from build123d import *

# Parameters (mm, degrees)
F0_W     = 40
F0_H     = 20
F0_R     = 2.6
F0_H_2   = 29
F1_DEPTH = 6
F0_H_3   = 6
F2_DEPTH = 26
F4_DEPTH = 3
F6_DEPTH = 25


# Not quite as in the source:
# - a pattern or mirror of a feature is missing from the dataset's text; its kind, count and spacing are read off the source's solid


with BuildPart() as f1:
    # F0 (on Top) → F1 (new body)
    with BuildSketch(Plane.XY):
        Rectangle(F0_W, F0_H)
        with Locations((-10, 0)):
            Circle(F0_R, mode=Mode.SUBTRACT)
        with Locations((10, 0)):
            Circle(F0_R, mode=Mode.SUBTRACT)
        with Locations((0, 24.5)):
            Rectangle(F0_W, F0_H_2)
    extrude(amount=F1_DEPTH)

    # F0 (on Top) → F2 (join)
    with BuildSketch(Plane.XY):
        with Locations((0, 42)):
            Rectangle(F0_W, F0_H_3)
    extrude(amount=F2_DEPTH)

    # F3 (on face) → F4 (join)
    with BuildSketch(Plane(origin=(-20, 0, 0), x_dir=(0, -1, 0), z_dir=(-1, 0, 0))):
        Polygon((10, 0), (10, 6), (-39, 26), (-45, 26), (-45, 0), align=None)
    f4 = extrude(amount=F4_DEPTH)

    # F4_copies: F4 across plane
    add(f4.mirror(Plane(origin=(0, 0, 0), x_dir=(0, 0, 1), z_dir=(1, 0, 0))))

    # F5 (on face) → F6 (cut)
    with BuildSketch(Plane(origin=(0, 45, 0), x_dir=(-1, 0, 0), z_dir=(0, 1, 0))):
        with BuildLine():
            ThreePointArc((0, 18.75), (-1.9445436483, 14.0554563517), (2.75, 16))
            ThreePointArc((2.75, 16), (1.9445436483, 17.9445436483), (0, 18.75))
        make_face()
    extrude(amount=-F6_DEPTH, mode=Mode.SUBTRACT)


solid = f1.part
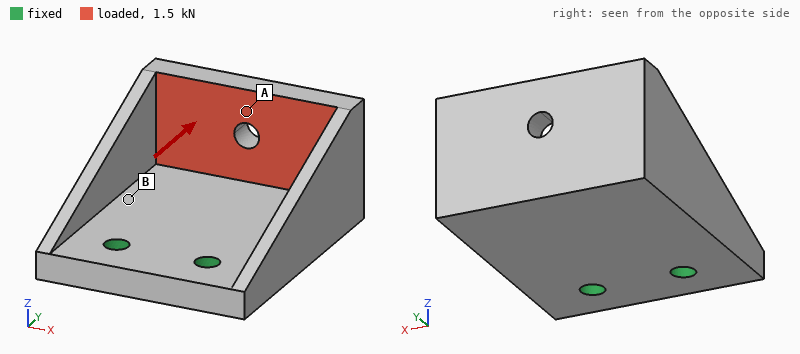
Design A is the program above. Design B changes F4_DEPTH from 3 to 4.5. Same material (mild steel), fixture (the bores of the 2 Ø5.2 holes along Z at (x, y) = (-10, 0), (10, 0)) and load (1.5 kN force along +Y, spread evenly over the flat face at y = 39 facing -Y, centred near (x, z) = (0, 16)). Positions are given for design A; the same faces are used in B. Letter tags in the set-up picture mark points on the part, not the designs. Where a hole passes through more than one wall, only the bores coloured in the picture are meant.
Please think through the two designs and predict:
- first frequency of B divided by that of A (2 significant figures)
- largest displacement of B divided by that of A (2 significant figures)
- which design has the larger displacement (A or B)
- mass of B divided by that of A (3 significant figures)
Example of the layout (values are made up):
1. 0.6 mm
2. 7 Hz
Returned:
1. 0.98
2. 0.90
3. A
4. 1.12
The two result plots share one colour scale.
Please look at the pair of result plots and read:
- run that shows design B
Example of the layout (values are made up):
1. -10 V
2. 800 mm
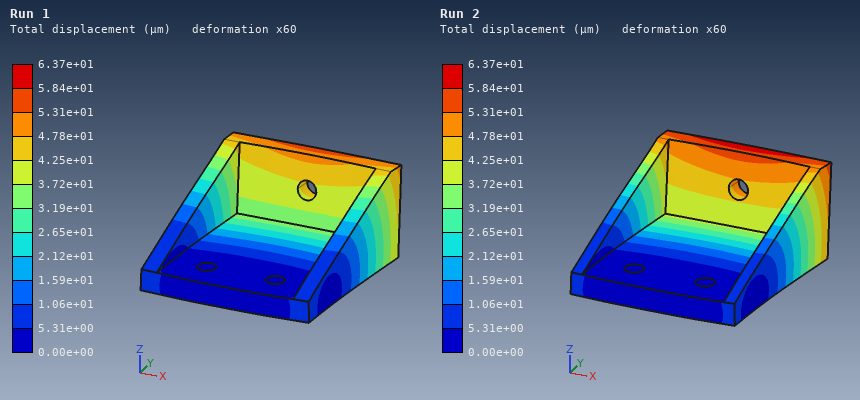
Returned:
1. Run 1
